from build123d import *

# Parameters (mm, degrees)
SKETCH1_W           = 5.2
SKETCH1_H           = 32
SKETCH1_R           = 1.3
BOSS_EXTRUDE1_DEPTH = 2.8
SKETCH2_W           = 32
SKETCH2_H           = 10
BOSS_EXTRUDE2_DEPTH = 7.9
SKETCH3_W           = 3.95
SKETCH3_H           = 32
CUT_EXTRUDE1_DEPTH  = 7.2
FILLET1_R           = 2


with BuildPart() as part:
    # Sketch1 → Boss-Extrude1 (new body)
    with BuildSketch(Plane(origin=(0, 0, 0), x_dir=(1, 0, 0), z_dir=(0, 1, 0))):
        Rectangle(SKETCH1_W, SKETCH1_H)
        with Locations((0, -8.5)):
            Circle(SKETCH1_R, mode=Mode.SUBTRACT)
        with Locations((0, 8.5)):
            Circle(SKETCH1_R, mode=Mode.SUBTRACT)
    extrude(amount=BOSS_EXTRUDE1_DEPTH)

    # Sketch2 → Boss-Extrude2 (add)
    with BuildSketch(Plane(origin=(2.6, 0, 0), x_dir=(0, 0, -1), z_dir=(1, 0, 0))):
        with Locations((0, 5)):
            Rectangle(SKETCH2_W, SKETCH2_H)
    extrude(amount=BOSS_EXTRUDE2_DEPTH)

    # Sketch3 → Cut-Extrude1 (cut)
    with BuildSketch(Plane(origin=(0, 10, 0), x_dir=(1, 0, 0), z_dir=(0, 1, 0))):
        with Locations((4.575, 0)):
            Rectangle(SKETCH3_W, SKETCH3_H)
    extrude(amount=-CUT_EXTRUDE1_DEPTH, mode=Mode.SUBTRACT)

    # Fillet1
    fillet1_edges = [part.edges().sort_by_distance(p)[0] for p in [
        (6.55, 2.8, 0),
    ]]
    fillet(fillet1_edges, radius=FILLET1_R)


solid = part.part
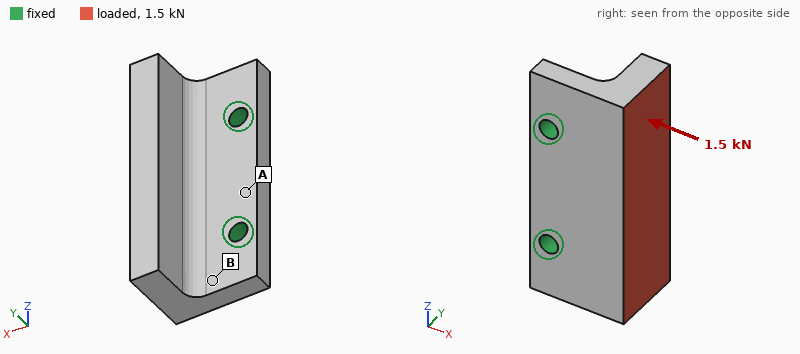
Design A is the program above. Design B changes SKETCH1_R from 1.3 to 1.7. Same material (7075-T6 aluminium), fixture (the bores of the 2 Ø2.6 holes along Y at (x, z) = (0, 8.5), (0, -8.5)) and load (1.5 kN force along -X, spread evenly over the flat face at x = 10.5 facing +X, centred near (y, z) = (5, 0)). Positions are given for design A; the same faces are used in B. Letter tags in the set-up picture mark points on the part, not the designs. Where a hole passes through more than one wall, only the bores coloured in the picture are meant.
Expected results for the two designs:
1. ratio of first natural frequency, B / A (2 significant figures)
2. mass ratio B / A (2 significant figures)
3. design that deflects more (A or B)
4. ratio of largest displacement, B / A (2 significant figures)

1.1
0.99
A
0.88
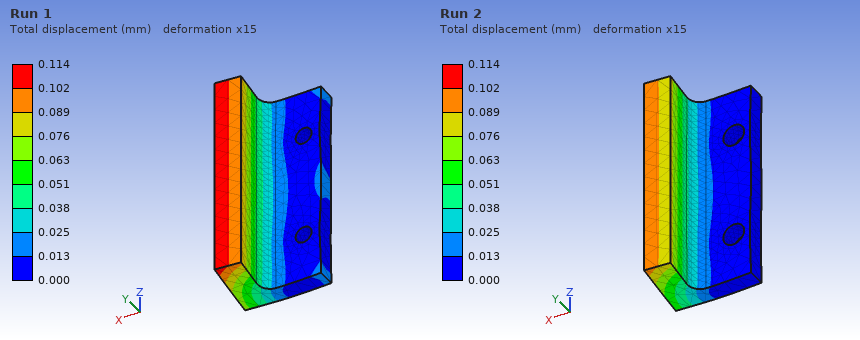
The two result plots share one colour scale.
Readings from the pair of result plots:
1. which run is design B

Run 2
